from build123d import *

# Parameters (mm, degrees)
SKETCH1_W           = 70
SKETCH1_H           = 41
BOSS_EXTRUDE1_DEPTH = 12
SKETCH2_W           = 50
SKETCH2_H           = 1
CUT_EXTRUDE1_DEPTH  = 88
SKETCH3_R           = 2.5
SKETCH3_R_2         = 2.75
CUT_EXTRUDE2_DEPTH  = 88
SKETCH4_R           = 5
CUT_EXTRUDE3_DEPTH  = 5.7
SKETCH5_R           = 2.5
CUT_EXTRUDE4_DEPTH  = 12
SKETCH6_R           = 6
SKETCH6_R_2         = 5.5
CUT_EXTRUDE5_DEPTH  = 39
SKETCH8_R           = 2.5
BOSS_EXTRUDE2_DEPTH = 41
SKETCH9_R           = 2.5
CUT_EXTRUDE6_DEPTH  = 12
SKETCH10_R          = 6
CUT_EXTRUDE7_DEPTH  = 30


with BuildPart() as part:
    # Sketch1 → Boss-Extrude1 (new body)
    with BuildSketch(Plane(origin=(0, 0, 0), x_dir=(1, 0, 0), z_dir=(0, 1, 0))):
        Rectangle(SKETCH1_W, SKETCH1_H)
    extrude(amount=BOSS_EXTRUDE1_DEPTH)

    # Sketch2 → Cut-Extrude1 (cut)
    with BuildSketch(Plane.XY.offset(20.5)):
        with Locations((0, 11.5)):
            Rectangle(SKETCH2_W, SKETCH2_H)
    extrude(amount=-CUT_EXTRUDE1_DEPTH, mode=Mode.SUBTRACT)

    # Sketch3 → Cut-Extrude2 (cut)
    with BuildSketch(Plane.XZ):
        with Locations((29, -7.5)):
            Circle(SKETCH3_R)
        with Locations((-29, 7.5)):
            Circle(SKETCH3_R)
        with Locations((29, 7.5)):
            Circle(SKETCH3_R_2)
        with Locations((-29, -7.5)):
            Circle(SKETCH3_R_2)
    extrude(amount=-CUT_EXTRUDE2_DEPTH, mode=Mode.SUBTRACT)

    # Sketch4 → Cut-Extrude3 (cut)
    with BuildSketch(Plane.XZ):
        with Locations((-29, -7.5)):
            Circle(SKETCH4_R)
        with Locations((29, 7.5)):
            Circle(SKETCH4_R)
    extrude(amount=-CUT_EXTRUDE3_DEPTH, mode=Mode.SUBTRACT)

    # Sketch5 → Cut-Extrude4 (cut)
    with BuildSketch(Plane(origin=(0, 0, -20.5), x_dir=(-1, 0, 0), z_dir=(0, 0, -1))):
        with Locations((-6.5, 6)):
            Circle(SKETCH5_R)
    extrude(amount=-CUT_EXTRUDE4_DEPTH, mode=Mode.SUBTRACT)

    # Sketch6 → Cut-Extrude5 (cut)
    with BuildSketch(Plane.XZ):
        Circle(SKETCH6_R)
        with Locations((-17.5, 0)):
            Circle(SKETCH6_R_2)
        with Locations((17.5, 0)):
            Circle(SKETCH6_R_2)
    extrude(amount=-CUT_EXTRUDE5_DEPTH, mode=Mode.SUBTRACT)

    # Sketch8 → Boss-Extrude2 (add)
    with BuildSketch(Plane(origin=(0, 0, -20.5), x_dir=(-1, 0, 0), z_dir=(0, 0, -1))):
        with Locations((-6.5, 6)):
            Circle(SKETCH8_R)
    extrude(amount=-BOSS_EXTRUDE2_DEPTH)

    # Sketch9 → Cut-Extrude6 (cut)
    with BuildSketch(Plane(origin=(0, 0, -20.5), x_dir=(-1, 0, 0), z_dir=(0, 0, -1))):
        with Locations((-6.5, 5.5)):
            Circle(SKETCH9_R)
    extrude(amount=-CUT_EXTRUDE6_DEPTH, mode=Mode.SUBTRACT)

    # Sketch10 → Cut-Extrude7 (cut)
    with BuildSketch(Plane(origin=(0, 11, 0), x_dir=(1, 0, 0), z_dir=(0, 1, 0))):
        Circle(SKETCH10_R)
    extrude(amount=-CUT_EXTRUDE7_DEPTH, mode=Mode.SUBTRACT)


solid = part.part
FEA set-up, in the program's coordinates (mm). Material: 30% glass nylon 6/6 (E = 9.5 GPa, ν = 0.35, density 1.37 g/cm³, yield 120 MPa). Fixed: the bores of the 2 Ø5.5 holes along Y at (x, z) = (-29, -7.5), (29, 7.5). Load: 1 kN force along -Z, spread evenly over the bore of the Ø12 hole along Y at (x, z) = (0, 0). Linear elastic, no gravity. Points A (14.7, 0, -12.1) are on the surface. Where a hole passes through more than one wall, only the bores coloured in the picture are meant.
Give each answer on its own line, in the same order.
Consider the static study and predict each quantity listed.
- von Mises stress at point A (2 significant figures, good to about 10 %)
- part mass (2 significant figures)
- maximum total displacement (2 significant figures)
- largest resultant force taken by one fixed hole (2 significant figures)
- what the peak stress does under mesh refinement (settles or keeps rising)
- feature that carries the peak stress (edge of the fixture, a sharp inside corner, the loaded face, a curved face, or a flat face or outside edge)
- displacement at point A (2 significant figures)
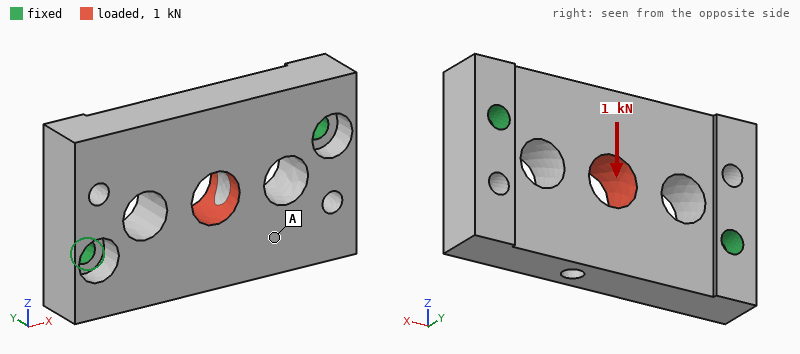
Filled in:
3.0 MPa
37 g
44 µm
510 N
keeps rising
edge of the fixture
34 µm
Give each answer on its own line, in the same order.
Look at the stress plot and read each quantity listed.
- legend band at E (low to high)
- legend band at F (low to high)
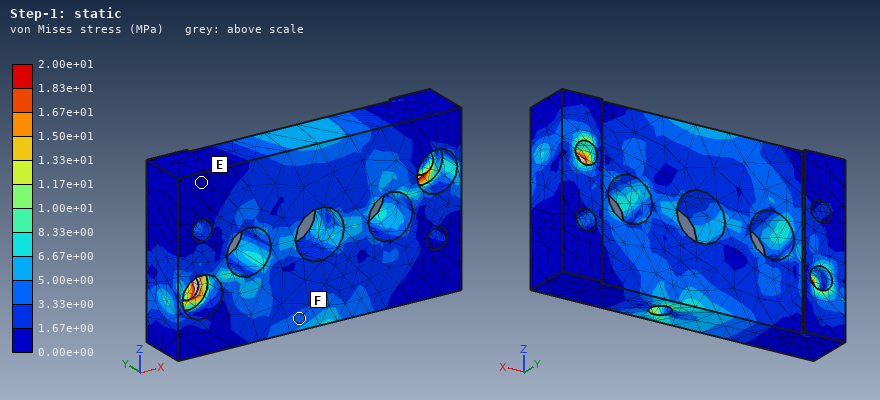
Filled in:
0.00e+00 to 1.67e+00 MPa
3.33e+00 to 5.00e+00 MPa
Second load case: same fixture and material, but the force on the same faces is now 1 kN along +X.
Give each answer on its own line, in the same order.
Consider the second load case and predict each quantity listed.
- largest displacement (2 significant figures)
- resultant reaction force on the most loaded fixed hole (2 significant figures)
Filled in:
17 µm
510 N
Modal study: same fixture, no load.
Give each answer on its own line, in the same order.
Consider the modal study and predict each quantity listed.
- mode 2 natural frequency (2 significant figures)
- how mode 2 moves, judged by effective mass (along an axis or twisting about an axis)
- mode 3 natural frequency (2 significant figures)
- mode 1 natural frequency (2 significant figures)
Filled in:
3900 Hz
along Y
6300 Hz
2800 Hz
